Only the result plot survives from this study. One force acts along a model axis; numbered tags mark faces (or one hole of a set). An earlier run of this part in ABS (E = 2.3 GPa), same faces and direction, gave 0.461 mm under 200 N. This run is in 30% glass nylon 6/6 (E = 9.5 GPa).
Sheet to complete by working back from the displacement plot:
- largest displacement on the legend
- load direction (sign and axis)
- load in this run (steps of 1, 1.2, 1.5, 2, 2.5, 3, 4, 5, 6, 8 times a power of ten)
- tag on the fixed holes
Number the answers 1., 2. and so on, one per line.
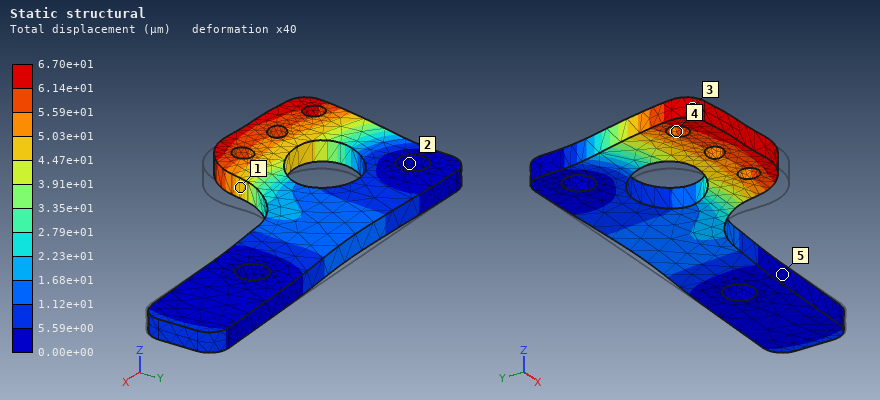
1. 6.70e+01 µm
2. -X
3. 120 N
4. 2
